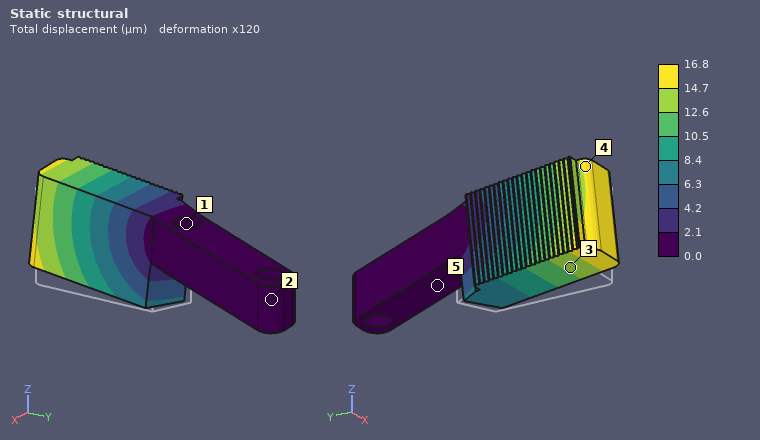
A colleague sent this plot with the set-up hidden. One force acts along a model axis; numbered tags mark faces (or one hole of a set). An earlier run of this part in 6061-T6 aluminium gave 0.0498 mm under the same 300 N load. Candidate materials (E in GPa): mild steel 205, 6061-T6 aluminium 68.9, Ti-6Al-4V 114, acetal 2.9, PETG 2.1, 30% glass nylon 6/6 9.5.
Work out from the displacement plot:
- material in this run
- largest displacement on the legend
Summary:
mild steel
16.8 µm
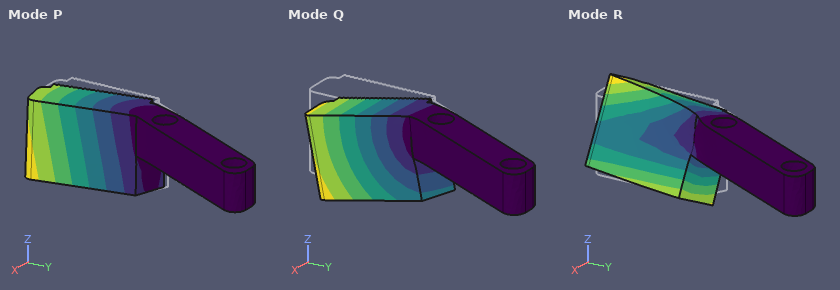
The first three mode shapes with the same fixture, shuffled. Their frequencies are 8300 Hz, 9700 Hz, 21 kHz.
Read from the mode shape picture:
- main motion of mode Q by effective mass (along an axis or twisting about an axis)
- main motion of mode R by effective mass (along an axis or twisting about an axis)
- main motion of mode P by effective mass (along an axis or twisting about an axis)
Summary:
along Z
twisting about Y
along X
